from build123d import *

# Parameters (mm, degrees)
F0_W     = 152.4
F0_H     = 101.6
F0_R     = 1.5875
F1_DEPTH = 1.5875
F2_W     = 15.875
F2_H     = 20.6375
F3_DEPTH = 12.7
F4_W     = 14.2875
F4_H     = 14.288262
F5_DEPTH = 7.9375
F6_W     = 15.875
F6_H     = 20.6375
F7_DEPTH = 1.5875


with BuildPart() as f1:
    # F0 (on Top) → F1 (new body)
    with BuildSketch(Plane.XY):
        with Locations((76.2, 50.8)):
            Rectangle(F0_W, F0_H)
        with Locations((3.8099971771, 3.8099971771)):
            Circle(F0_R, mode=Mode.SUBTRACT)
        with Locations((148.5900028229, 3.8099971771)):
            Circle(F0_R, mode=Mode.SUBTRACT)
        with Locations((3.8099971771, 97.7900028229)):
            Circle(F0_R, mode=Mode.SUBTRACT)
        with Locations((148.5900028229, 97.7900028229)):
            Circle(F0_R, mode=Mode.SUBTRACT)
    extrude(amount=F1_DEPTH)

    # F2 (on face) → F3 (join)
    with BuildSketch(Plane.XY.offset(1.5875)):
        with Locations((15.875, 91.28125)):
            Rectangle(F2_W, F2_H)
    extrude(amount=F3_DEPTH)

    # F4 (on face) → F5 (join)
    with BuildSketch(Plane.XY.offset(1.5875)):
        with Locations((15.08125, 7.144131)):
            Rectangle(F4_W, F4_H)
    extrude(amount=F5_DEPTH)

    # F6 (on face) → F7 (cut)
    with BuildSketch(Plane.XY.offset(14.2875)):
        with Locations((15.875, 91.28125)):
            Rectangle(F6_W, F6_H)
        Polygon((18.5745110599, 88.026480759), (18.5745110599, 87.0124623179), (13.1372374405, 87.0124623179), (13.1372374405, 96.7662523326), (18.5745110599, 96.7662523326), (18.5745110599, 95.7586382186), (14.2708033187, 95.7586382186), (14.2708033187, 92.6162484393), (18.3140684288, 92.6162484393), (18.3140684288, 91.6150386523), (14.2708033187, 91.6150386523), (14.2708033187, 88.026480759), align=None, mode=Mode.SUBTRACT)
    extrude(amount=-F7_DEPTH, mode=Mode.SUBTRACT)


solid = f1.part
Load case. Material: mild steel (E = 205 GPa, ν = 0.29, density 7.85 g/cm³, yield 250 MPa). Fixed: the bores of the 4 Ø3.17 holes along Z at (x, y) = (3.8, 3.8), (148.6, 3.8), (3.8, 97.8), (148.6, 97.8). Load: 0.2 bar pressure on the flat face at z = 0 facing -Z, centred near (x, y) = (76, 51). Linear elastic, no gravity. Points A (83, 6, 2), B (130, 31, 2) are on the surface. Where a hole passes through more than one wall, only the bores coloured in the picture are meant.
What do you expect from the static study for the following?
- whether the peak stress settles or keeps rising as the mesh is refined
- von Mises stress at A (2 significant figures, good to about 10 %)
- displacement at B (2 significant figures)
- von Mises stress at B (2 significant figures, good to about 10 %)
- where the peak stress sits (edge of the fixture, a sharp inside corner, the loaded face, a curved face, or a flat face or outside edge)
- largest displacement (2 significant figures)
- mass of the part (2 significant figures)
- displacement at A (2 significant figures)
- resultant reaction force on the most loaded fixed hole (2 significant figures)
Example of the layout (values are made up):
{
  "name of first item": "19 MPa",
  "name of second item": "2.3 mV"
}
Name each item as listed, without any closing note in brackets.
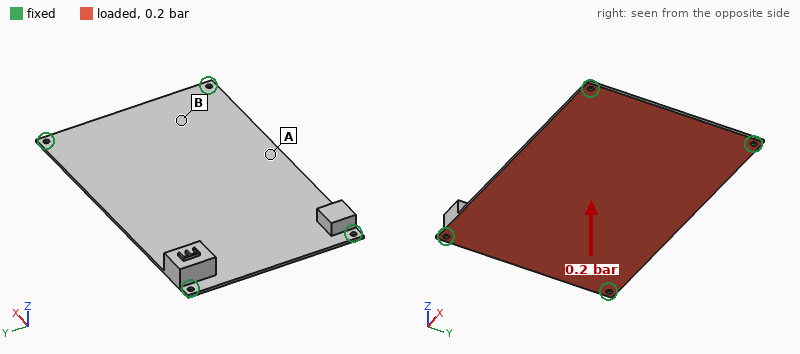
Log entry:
{
  "whether the peak stress settles or keeps rising as the mesh is refined": "keeps rising",
  "von Mises stress at A": "54 MPa",
  "displacement at B": "0.23 mm",
  "von Mises stress at B": "22 MPa",
  "where the peak stress sits": "edge of the fixture",
  "largest displacement": "0.55 mm",
  "mass of the part": "230 g",
  "displacement at A": "0.50 mm",
  "resultant reaction force on the most loaded fixed hole": "89 N"
}
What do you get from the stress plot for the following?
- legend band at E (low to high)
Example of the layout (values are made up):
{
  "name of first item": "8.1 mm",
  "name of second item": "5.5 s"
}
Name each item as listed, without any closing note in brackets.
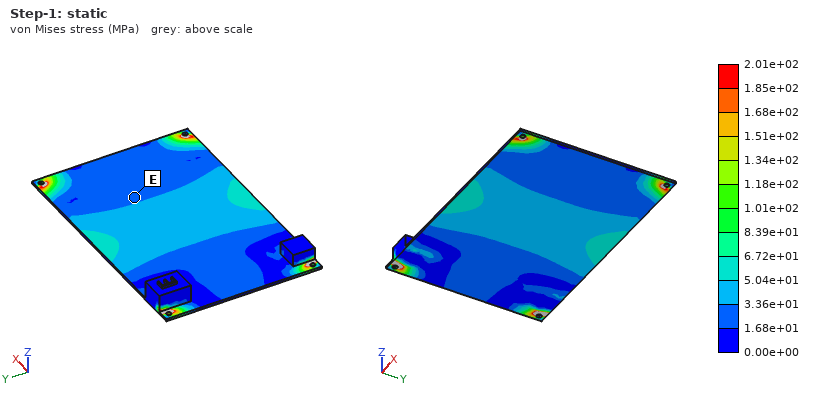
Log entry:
{
  "legend band at E": "1.68e+01 to 3.36e+01 MPa"
}
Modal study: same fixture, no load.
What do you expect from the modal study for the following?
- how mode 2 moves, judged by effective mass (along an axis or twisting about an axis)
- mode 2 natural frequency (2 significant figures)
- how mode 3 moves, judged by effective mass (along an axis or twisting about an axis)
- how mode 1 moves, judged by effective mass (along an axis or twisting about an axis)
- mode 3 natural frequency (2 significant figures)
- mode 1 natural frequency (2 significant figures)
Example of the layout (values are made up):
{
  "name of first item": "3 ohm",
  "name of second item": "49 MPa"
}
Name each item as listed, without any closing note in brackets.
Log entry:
{
  "how mode 2 moves, judged by effective mass": "twisting about X",
  "mode 2 natural frequency": "560 Hz",
  "how mode 3 moves, judged by effective mass": "twisting about Y",
  "how mode 1 moves, judged by effective mass": "along Z",
  "mode 3 natural frequency": "760 Hz",
  "mode 1 natural frequency": "310 Hz"
}
